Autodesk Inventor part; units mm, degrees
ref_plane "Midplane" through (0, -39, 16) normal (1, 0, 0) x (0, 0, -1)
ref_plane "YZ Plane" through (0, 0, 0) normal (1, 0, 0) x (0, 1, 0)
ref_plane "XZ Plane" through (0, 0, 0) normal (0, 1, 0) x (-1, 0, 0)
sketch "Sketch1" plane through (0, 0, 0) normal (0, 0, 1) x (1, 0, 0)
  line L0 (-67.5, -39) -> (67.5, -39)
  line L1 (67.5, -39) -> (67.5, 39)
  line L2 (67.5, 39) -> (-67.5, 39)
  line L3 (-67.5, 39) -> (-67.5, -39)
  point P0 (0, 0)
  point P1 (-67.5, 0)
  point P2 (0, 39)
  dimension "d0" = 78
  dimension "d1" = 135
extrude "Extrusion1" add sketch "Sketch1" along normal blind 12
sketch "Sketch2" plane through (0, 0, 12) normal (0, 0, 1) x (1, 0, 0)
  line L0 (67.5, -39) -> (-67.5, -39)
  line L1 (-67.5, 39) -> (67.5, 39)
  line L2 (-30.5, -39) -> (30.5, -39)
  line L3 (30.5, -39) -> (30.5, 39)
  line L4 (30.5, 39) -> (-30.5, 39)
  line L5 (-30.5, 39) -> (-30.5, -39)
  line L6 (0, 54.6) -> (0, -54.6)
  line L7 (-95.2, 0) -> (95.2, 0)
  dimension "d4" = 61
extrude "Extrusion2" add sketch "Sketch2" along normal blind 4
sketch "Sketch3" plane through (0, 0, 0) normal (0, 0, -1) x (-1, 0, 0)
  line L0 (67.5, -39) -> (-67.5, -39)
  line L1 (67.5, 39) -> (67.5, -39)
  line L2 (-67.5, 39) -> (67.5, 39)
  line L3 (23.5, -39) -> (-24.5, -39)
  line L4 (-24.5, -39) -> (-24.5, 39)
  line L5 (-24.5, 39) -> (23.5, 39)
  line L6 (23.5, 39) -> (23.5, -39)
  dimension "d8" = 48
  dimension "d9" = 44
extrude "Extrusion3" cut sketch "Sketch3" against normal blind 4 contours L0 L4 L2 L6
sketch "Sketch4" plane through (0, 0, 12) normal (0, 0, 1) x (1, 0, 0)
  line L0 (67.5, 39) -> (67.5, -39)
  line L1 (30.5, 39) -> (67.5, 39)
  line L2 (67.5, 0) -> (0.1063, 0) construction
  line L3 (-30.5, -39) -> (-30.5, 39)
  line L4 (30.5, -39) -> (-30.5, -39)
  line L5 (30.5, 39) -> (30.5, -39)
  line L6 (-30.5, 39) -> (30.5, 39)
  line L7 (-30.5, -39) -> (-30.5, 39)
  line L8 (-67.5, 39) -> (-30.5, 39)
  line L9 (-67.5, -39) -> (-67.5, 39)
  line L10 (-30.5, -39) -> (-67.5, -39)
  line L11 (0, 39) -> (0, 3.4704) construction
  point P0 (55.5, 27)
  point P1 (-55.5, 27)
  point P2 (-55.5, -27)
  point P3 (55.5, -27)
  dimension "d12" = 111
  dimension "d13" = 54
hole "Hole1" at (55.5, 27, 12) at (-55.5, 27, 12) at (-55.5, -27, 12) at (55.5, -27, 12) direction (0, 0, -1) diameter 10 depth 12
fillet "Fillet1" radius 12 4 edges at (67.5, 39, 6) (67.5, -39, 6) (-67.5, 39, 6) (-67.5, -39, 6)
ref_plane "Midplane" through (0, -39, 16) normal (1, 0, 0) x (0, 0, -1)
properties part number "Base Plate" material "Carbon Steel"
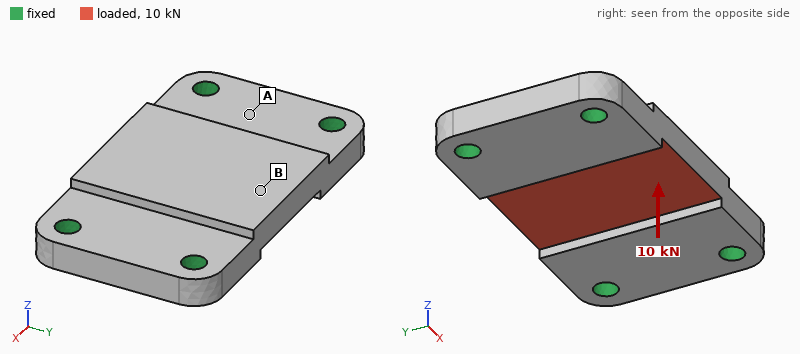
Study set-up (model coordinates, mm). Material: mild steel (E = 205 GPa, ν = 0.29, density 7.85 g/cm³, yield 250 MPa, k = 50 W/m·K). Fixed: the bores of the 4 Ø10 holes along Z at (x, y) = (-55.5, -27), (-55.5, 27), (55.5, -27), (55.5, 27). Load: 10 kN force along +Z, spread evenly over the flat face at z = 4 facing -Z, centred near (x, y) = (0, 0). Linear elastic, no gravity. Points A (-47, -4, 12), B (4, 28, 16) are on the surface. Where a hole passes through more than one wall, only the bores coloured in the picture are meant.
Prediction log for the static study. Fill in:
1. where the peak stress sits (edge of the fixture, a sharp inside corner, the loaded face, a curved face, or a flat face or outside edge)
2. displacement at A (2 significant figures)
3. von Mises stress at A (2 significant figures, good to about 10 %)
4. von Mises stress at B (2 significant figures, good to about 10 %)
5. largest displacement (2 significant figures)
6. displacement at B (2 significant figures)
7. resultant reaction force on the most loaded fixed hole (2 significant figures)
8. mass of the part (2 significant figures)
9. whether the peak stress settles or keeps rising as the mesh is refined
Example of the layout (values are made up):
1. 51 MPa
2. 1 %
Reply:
1. edge of the fixture
2. 4.2 µm
3. 17 MPa
4. 45 MPa
5. 26 µm
6. 24 µm
7. 4.3 kN
8. 980 g
9. keeps rising
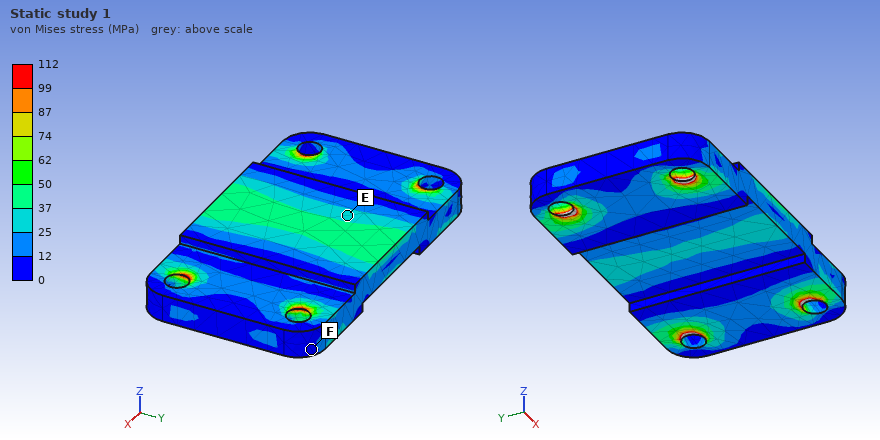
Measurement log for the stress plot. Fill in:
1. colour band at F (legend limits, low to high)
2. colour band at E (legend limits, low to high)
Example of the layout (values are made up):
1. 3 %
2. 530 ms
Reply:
1. 0 to 12 MPa
2. 25 to 37 MPa
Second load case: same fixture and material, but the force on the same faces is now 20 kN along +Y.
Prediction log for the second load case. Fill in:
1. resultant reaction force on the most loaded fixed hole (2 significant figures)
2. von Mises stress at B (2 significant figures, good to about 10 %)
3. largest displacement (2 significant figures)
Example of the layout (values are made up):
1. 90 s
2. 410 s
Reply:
1. 6.2 kN
2. 19 MPa
3. 12 µm
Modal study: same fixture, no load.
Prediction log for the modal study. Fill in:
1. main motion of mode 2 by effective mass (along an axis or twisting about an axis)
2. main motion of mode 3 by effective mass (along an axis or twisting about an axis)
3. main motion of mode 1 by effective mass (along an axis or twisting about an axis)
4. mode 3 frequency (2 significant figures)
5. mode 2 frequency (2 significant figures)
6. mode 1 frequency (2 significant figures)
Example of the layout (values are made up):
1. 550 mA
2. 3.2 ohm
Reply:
1. twisting about X
2. twisting about Y
3. along Z
4. 11 kHz
5. 6900 Hz
6. 5100 Hz
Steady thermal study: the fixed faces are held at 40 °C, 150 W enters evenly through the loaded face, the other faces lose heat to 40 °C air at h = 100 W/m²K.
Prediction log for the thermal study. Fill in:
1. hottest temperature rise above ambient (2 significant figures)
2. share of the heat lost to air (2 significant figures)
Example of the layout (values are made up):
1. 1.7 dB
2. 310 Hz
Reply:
1. 58 K
2. 34 %
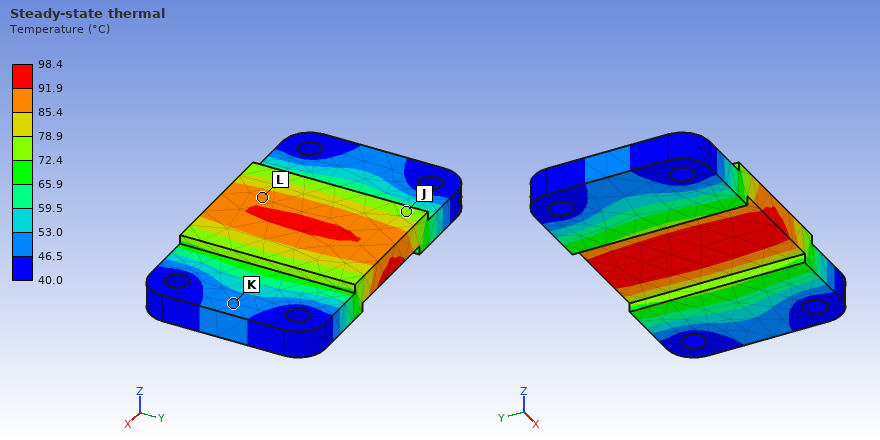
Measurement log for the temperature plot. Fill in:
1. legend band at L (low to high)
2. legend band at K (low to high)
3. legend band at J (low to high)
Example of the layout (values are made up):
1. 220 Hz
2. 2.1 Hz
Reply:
1. 85.4 to 91.9 °C
2. 46.5 to 53.0 °C
3. 72.4 to 78.9 °C
